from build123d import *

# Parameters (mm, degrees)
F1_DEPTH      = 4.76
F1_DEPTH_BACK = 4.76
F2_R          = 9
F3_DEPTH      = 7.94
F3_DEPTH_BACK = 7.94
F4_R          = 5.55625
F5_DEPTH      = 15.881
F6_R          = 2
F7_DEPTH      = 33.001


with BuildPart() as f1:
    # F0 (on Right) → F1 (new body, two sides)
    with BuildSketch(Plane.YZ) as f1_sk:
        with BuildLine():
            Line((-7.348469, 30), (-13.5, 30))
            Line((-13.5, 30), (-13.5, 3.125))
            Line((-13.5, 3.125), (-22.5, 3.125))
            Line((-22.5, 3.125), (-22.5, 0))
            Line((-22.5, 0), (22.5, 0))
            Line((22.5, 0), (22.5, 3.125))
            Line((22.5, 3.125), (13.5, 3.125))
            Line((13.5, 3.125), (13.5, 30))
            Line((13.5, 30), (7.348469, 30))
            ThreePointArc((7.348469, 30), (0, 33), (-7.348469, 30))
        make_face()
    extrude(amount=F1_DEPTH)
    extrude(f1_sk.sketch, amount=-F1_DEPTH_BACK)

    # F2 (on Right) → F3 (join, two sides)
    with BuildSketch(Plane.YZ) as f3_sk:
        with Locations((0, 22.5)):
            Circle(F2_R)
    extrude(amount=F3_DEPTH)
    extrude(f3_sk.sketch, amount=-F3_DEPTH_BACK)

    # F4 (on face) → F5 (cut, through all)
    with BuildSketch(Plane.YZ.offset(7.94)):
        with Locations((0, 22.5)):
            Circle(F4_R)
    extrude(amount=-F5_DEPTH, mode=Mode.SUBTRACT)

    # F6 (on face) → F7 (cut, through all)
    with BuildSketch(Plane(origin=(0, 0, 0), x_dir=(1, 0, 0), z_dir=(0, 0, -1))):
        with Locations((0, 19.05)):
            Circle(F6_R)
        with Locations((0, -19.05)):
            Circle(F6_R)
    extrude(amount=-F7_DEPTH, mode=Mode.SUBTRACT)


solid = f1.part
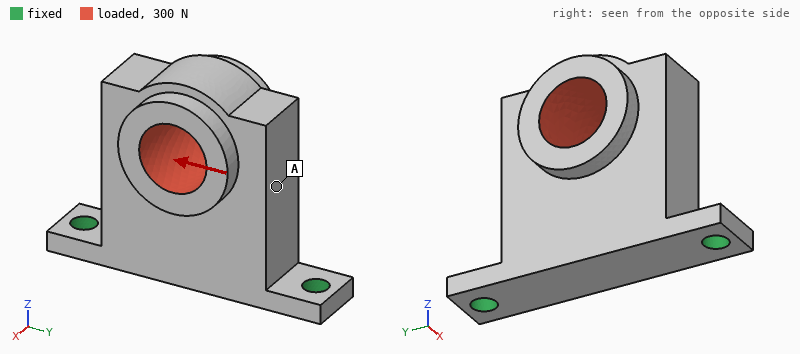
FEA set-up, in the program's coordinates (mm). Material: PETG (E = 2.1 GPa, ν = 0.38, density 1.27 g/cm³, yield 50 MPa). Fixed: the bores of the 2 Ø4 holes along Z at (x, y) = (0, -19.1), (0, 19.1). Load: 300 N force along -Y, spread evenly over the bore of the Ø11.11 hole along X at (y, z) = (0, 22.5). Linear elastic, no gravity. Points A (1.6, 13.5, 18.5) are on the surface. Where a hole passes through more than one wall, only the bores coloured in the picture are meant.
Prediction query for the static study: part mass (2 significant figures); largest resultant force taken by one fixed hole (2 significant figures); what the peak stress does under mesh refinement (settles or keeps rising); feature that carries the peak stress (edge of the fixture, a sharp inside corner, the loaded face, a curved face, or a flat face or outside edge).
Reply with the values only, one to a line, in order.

11 g
250 N
keeps rising
edge of the fixture
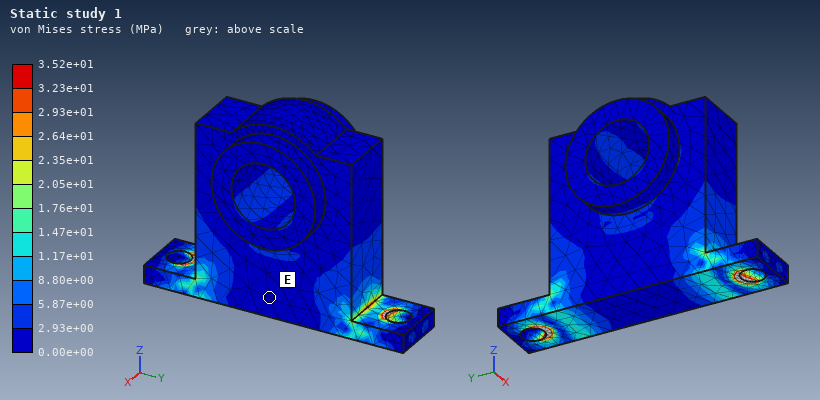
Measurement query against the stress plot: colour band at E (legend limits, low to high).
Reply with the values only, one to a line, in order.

0.00e+00 to 2.93e+00 MPa
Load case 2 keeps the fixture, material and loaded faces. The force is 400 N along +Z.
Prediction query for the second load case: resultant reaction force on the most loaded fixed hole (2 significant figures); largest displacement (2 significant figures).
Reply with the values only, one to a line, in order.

230 N
0.17 mm
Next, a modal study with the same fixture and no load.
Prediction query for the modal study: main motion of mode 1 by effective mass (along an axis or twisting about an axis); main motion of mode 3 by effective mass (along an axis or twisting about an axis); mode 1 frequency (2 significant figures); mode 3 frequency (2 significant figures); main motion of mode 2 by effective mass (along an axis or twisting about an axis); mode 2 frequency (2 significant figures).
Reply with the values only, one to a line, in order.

along X
along Z
490 Hz
2600 Hz
along Y
2000 Hz
